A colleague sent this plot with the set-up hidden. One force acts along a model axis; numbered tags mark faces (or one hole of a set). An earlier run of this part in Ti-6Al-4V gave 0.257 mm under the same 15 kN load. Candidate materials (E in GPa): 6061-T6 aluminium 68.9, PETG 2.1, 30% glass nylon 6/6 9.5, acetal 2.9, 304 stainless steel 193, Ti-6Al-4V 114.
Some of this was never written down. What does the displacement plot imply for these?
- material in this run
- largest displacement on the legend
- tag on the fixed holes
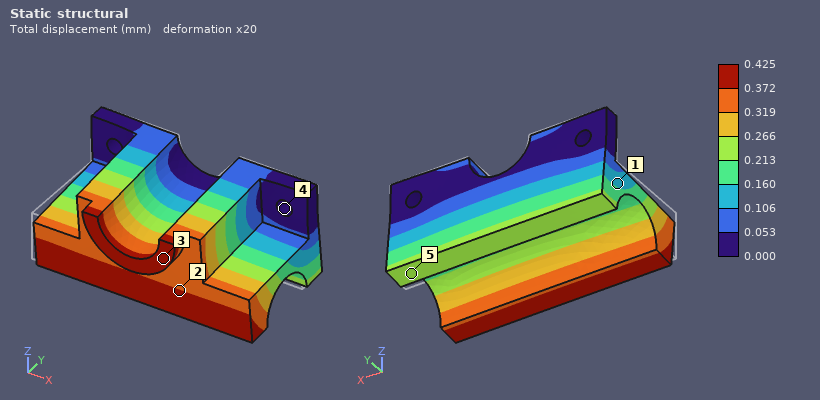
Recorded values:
6061-T6 aluminium
0.425 mm
4
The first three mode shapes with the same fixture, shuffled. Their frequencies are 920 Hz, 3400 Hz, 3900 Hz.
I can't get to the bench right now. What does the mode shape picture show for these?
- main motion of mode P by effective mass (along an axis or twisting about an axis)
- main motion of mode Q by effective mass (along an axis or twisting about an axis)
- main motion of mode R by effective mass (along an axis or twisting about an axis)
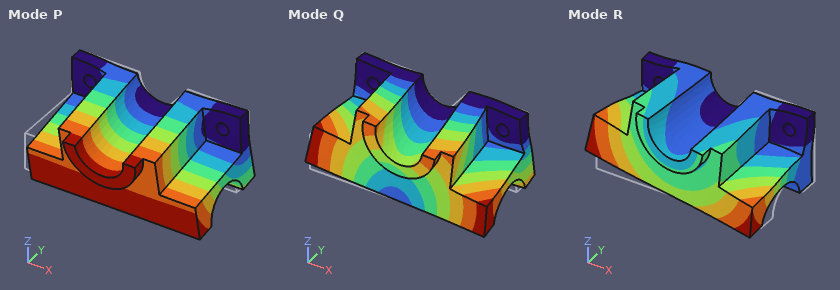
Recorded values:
along Z
along X
along X
